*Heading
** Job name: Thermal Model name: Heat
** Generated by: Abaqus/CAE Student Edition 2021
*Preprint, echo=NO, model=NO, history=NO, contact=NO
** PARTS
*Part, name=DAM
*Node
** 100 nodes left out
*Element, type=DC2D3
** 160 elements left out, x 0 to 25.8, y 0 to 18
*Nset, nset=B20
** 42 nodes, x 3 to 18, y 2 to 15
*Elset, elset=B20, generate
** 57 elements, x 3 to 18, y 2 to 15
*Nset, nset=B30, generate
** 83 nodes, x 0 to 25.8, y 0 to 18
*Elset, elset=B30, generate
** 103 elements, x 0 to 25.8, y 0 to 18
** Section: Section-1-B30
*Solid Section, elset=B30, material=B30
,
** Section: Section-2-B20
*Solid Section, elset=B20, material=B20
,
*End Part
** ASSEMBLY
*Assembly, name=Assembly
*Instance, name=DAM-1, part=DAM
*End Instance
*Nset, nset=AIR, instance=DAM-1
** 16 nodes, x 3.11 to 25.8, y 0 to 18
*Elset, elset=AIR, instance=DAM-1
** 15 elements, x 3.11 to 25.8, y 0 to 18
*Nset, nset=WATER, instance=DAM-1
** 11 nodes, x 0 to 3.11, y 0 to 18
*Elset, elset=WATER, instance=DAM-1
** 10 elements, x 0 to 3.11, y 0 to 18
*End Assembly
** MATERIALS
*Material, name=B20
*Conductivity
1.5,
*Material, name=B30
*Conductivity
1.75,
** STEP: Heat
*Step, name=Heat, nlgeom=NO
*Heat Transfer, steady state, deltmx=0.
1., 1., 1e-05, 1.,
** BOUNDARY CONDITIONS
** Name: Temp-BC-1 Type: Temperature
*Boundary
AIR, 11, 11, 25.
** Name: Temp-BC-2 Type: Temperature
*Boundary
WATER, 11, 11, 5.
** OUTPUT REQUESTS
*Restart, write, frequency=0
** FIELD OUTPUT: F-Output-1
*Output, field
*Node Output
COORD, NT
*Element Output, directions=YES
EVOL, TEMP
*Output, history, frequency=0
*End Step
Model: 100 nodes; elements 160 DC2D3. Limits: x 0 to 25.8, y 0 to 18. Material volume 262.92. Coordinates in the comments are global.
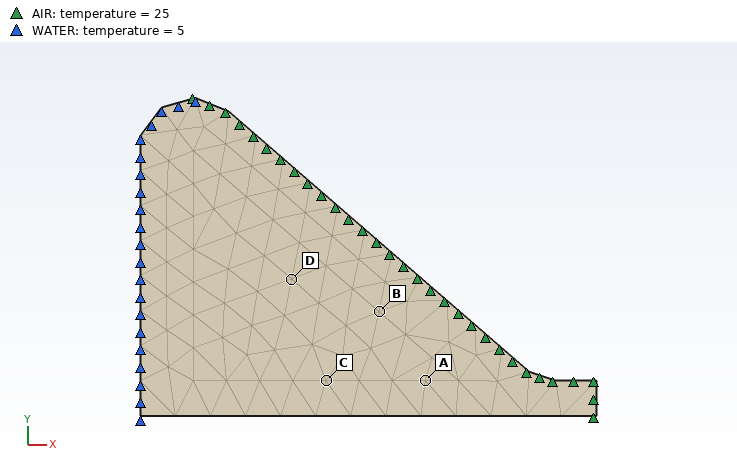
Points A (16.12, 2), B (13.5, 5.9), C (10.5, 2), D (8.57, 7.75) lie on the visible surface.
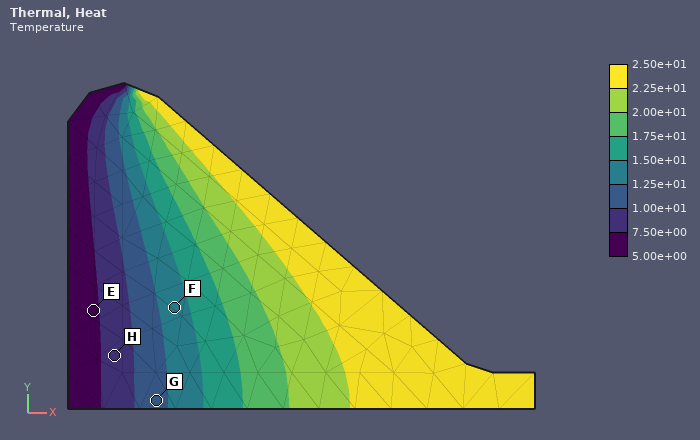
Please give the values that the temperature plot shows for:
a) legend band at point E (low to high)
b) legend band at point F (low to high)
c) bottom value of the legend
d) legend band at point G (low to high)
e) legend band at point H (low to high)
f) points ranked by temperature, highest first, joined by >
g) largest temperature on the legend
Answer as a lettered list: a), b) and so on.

a) 5.00e+00 to 7.50e+00
b) 1.25e+01 to 1.50e+01
c) 5.00e+00
d) 1.00e+01 to 1.25e+01
e) 7.50e+00 to 1.00e+01
f) F > G > H > E
g) 2.50e+01
